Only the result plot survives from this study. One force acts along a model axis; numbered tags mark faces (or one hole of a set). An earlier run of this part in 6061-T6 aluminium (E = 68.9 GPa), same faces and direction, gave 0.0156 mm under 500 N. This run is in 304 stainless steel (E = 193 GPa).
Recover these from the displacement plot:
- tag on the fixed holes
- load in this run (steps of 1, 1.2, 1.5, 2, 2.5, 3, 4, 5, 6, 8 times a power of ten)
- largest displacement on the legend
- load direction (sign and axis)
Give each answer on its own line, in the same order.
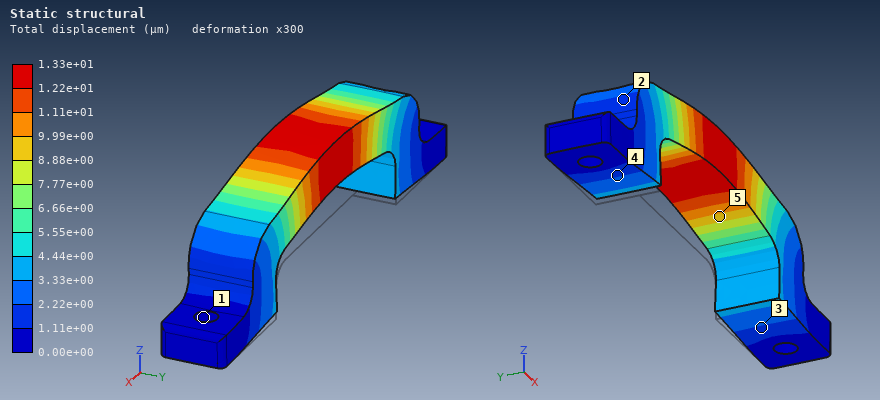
1
1.2 kN
1.33e+01 µm
+Z
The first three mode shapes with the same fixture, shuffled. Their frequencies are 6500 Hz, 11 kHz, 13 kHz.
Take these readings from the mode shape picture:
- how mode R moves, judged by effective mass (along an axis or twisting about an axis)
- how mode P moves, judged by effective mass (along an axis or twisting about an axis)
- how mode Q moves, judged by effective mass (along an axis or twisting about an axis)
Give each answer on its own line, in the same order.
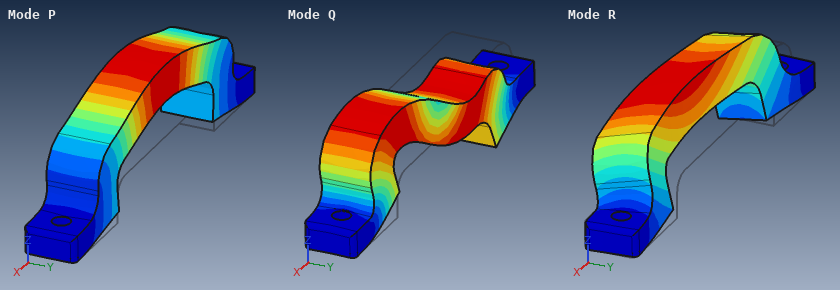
along Y
along Z
along X
